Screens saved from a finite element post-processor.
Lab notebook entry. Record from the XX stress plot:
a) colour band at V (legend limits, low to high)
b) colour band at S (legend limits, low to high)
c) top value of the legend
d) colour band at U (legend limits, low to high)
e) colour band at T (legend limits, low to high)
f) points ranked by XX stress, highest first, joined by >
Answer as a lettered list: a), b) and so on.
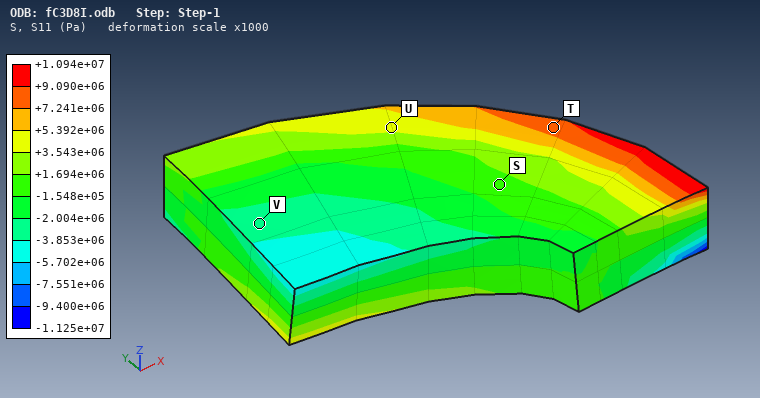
a) -3.853e+06 to -2.004e+06 Pa
b) -1.548e+05 to +1.694e+06 Pa
c) +1.094e+07 Pa
d) +3.543e+06 to +5.392e+06 Pa
e) +7.241e+06 to +9.090e+06 Pa
f) T > U > S > V
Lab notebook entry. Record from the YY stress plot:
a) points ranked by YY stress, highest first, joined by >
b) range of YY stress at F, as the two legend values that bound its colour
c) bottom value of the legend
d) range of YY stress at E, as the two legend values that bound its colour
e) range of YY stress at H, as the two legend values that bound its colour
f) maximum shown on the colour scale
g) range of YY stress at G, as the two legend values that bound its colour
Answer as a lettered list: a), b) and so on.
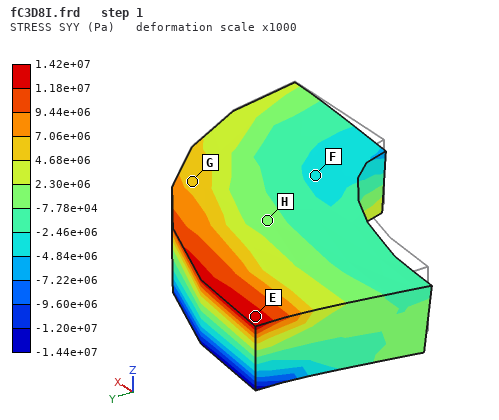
a) E > G > H > F
b) -4.84e+06 to -2.46e+06 Pa
c) -1.44e+07 Pa
d) 1.18e+07 to 1.42e+07 Pa
e) -7.78e+04 to 2.30e+06 Pa
f) 1.42e+07 Pa
g) 4.68e+06 to 7.06e+06 Pa
